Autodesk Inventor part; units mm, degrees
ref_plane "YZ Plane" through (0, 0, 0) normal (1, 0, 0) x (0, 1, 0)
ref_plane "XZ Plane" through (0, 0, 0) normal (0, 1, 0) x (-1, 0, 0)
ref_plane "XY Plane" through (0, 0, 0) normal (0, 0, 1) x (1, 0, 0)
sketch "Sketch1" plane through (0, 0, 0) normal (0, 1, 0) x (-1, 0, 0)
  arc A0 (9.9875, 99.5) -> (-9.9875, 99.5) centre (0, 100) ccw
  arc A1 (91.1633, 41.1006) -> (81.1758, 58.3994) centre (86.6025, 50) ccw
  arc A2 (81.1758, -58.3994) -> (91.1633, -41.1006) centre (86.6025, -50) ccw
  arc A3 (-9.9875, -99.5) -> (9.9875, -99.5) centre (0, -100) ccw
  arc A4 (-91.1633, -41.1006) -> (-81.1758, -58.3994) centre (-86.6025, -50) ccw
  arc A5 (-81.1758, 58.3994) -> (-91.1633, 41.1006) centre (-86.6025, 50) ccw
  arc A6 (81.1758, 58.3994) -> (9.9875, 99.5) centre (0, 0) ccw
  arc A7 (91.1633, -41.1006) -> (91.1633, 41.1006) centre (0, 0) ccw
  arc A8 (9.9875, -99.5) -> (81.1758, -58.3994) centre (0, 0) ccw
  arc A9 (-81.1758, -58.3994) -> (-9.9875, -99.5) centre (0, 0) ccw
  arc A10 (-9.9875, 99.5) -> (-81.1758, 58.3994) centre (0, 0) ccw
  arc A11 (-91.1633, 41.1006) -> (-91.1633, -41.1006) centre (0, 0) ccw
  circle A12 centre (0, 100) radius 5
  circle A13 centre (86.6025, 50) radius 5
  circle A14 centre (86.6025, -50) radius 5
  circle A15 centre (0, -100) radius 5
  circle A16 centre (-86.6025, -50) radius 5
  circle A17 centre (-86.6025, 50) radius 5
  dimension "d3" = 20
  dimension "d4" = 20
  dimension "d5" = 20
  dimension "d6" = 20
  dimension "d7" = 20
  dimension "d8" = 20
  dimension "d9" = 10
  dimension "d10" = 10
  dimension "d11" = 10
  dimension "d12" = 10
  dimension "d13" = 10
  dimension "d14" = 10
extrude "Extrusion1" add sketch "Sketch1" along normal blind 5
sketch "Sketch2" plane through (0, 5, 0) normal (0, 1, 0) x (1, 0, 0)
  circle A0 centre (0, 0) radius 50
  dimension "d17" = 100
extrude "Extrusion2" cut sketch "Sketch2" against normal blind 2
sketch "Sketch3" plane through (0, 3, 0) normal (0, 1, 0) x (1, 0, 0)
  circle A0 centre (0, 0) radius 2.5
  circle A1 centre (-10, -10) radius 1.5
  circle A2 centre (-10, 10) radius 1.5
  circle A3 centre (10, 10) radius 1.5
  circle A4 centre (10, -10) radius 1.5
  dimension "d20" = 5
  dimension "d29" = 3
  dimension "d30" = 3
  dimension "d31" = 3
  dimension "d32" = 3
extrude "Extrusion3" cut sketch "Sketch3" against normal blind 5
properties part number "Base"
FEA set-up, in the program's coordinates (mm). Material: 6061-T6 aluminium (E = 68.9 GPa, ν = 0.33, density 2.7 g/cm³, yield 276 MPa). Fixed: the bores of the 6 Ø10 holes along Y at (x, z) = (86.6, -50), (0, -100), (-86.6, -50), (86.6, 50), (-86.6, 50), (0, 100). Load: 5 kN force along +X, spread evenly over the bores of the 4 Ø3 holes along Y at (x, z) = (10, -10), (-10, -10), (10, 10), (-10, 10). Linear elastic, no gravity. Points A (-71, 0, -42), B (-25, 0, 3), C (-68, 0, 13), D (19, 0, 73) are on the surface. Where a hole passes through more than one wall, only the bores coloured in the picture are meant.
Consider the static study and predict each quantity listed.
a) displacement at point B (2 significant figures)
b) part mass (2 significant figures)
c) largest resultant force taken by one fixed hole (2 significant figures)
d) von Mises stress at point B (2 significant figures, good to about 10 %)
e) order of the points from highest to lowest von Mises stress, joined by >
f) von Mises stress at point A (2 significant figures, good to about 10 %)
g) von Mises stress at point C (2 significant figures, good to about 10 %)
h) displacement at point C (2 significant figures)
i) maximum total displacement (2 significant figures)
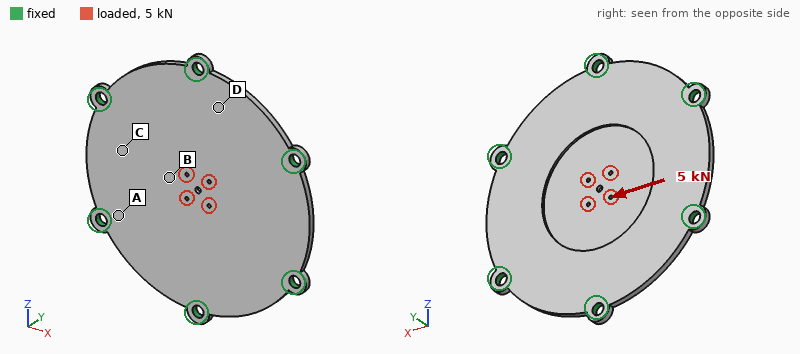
14 µm
390 g
1.1 kN
12 MPa
B > A > C > D
9.8 MPa
4.9 MPa
5.6 µm
17 µm
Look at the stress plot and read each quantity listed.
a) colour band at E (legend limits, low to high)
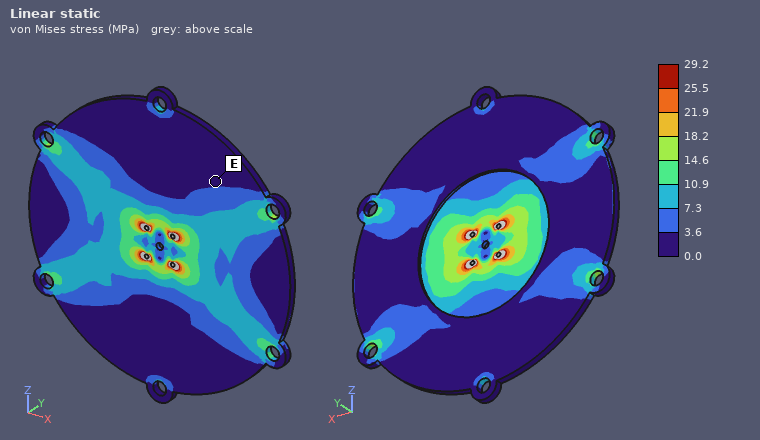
0.0 to 3.6 MPa
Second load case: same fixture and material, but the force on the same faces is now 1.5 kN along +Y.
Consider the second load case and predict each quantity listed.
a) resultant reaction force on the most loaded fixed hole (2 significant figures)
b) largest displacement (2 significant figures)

970 N
0.89 mm
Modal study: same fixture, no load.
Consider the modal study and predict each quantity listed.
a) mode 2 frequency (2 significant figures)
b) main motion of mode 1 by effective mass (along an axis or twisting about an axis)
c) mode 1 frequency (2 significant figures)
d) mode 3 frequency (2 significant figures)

1900 Hz
along Y
1000 Hz
1900 Hz
